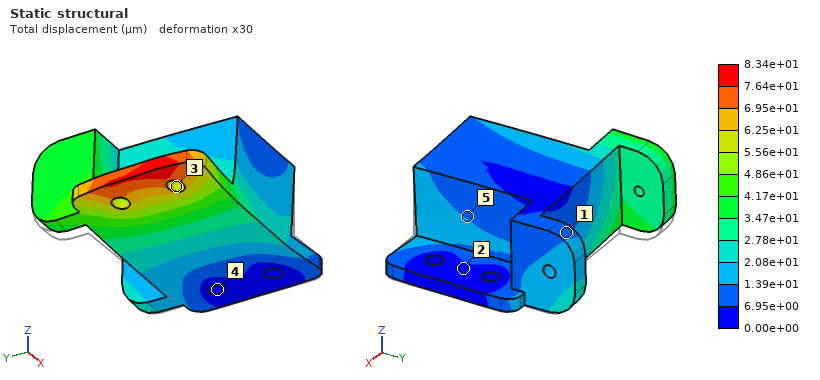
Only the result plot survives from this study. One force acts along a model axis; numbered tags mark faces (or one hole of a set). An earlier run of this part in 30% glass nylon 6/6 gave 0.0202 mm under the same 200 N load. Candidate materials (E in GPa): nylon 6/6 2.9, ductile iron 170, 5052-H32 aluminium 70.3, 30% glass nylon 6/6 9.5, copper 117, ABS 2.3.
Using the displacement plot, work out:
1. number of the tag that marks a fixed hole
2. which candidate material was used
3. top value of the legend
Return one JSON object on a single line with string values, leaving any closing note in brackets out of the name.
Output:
{"number of the tag that marks a fixed hole": "4", "which candidate material was used": "ABS", "top value of the legend": "8.34e+01 µm"}
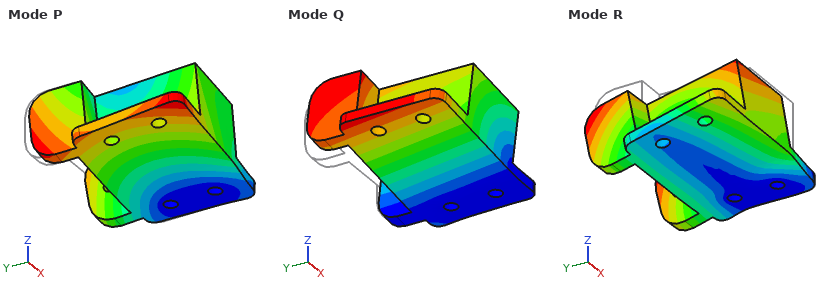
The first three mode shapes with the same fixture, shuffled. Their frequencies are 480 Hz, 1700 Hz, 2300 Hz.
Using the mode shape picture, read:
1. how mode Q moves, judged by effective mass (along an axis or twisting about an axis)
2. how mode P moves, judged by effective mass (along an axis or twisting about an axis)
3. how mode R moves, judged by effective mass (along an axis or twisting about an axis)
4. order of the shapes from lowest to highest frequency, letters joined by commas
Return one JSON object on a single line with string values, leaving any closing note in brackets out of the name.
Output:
{"how mode Q moves, judged by effective mass": "along Z", "how mode P moves, judged by effective mass": "along Y", "how mode R moves, judged by effective mass": "along Y", "order of the shapes from lowest to highest frequency, letters joined by commas": "Q, R, P"}
